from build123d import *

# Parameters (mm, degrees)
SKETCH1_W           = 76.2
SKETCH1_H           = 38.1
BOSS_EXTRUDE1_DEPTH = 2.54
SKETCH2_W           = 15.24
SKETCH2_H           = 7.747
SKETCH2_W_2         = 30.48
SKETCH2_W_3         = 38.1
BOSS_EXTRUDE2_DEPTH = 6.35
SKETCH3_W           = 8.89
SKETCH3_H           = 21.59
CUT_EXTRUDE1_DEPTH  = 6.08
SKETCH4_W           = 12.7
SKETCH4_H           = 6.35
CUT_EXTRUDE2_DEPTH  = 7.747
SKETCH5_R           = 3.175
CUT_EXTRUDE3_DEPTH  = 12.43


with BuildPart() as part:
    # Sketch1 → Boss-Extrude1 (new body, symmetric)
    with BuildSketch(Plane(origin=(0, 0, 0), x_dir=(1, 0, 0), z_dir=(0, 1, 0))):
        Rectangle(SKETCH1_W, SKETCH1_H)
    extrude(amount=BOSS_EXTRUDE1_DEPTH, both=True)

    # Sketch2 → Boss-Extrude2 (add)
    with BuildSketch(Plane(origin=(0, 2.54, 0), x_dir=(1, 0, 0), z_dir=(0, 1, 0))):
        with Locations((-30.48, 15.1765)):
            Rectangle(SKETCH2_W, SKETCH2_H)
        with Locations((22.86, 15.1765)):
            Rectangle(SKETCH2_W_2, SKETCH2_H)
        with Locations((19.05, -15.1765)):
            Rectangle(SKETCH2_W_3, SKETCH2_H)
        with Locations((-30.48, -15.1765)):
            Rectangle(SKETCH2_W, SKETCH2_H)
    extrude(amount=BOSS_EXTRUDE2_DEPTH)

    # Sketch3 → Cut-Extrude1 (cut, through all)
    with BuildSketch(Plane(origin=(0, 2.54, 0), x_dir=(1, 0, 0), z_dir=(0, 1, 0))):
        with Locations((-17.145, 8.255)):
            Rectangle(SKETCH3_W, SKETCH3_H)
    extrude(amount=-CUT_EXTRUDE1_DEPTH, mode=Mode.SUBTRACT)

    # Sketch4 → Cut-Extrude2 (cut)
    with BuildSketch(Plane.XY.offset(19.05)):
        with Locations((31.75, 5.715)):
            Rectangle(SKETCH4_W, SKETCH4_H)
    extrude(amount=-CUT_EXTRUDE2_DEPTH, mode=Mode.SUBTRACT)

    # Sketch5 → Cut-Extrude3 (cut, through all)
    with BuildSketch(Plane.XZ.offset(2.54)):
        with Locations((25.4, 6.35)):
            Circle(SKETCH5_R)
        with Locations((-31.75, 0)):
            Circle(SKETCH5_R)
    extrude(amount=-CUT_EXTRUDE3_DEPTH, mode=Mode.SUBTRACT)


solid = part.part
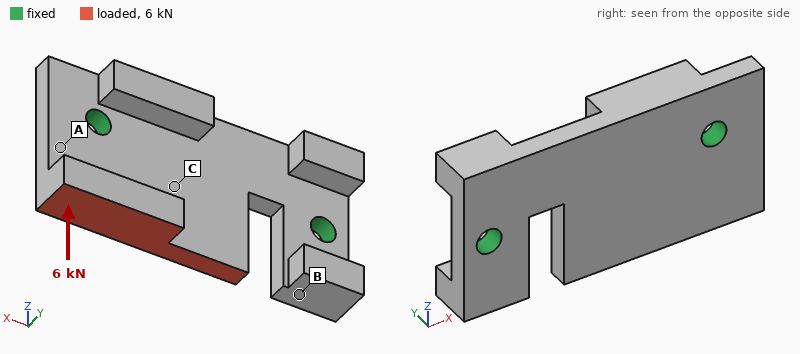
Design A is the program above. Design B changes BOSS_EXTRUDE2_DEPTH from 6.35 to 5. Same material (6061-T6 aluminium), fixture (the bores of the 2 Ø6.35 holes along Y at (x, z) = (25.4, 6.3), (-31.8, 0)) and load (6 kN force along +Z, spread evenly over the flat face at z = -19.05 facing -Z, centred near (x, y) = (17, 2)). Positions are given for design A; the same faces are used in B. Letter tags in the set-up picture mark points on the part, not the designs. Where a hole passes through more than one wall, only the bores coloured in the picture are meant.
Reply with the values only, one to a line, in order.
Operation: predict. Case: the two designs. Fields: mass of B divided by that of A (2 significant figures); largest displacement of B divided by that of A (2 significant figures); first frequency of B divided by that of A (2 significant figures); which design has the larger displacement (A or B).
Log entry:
0.95
0.75
1.0
A
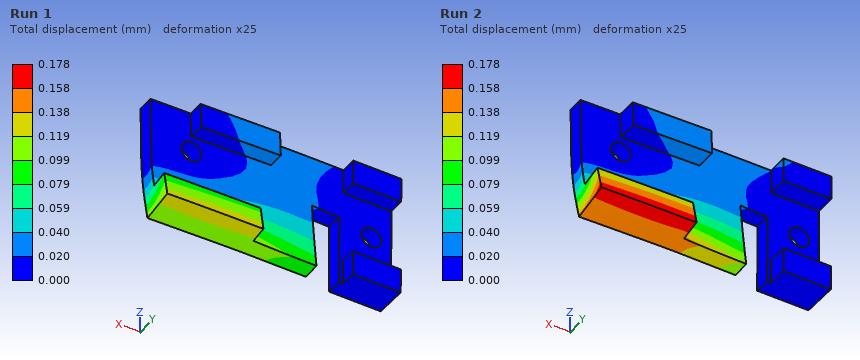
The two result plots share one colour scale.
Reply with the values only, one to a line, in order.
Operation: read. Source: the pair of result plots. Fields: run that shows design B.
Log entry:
Run 1
